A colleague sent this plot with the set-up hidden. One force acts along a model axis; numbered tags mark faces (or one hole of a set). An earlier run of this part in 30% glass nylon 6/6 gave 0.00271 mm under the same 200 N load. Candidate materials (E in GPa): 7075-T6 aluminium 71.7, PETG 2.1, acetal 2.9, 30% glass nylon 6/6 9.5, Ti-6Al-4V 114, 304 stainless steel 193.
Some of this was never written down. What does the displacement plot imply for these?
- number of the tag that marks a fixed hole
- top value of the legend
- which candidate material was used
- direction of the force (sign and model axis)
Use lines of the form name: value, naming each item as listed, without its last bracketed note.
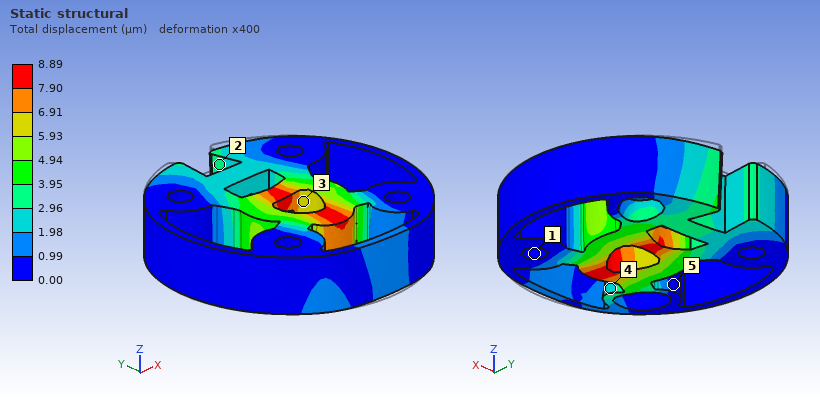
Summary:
number of the tag that marks a fixed hole: 1
top value of the legend: 8.89 µm
which candidate material was used: acetal
direction of the force: -Y
